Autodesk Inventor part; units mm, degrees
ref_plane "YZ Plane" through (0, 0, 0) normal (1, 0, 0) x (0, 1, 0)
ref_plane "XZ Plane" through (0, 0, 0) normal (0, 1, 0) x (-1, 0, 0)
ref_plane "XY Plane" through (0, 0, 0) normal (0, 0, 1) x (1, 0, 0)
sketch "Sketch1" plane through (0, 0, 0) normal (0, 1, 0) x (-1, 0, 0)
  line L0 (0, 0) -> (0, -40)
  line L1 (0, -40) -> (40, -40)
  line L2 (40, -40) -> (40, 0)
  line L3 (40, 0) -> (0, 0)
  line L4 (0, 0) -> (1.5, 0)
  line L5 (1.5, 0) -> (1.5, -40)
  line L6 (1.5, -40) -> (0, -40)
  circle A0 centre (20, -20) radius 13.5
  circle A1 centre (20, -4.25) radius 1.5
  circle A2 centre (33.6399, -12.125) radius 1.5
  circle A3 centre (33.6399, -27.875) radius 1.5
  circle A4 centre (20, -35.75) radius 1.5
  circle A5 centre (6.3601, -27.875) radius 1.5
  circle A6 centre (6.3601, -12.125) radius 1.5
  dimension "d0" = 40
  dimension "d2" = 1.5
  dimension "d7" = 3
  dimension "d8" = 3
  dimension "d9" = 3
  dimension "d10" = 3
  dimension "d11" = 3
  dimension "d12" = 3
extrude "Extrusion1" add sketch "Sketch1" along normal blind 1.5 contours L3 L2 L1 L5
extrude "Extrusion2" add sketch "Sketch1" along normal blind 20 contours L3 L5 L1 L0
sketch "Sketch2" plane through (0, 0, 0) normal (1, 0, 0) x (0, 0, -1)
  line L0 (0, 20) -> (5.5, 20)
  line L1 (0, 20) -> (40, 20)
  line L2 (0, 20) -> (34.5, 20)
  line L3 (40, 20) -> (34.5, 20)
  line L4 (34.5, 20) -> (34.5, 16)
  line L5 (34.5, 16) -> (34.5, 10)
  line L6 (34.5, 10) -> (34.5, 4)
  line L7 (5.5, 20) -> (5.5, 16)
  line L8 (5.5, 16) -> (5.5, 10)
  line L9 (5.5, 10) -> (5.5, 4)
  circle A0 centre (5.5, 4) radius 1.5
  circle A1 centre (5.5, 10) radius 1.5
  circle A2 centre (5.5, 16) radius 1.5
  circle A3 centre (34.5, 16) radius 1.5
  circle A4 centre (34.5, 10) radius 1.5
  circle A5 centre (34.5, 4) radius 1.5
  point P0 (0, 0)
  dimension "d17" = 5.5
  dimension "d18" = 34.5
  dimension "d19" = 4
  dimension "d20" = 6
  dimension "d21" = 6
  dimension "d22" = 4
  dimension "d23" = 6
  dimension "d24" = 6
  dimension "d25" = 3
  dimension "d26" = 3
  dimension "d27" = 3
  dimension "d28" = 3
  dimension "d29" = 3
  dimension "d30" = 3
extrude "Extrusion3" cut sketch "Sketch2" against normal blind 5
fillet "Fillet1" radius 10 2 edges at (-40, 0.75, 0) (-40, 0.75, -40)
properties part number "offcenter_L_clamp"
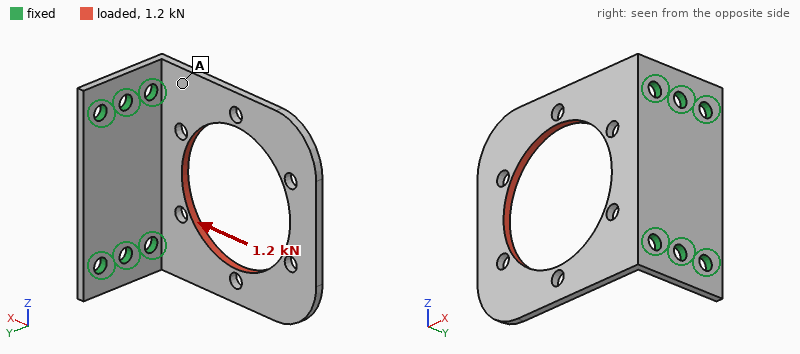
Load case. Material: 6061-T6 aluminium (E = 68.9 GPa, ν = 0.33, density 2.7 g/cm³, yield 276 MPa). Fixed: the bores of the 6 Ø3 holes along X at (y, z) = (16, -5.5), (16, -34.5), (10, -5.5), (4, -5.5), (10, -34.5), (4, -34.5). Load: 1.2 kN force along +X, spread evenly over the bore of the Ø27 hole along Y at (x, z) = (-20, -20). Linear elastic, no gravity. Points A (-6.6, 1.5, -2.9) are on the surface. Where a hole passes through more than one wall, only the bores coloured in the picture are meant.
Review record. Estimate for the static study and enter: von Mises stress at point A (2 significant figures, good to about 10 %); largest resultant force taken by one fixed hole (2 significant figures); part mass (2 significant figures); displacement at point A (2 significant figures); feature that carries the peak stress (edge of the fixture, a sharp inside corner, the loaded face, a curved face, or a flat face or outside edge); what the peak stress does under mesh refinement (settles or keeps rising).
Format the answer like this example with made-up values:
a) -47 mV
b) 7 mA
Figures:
a) 45 MPa
b) 650 N
c) 6.6 g
d) 0.050 mm
e) edge of the fixture
f) keeps rising
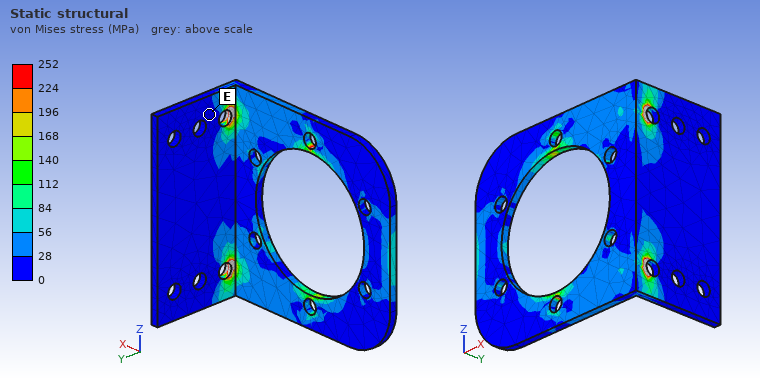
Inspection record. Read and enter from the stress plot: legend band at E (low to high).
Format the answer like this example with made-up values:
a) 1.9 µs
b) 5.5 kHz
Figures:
a) 0 to 28 MPa
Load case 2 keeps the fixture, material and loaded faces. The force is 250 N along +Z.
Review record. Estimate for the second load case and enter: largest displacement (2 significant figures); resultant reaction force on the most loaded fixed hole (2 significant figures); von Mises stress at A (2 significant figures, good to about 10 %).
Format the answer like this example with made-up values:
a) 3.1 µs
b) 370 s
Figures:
a) 71 µm
b) 180 N
c) 21 MPa
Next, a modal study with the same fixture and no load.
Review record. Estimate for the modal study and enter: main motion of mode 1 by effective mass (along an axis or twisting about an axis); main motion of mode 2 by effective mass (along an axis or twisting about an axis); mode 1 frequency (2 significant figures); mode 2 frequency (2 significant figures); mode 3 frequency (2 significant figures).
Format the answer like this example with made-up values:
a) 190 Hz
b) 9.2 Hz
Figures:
a) along Y
b) twisting about X
c) 640 Hz
d) 1600 Hz
e) 3900 Hz
